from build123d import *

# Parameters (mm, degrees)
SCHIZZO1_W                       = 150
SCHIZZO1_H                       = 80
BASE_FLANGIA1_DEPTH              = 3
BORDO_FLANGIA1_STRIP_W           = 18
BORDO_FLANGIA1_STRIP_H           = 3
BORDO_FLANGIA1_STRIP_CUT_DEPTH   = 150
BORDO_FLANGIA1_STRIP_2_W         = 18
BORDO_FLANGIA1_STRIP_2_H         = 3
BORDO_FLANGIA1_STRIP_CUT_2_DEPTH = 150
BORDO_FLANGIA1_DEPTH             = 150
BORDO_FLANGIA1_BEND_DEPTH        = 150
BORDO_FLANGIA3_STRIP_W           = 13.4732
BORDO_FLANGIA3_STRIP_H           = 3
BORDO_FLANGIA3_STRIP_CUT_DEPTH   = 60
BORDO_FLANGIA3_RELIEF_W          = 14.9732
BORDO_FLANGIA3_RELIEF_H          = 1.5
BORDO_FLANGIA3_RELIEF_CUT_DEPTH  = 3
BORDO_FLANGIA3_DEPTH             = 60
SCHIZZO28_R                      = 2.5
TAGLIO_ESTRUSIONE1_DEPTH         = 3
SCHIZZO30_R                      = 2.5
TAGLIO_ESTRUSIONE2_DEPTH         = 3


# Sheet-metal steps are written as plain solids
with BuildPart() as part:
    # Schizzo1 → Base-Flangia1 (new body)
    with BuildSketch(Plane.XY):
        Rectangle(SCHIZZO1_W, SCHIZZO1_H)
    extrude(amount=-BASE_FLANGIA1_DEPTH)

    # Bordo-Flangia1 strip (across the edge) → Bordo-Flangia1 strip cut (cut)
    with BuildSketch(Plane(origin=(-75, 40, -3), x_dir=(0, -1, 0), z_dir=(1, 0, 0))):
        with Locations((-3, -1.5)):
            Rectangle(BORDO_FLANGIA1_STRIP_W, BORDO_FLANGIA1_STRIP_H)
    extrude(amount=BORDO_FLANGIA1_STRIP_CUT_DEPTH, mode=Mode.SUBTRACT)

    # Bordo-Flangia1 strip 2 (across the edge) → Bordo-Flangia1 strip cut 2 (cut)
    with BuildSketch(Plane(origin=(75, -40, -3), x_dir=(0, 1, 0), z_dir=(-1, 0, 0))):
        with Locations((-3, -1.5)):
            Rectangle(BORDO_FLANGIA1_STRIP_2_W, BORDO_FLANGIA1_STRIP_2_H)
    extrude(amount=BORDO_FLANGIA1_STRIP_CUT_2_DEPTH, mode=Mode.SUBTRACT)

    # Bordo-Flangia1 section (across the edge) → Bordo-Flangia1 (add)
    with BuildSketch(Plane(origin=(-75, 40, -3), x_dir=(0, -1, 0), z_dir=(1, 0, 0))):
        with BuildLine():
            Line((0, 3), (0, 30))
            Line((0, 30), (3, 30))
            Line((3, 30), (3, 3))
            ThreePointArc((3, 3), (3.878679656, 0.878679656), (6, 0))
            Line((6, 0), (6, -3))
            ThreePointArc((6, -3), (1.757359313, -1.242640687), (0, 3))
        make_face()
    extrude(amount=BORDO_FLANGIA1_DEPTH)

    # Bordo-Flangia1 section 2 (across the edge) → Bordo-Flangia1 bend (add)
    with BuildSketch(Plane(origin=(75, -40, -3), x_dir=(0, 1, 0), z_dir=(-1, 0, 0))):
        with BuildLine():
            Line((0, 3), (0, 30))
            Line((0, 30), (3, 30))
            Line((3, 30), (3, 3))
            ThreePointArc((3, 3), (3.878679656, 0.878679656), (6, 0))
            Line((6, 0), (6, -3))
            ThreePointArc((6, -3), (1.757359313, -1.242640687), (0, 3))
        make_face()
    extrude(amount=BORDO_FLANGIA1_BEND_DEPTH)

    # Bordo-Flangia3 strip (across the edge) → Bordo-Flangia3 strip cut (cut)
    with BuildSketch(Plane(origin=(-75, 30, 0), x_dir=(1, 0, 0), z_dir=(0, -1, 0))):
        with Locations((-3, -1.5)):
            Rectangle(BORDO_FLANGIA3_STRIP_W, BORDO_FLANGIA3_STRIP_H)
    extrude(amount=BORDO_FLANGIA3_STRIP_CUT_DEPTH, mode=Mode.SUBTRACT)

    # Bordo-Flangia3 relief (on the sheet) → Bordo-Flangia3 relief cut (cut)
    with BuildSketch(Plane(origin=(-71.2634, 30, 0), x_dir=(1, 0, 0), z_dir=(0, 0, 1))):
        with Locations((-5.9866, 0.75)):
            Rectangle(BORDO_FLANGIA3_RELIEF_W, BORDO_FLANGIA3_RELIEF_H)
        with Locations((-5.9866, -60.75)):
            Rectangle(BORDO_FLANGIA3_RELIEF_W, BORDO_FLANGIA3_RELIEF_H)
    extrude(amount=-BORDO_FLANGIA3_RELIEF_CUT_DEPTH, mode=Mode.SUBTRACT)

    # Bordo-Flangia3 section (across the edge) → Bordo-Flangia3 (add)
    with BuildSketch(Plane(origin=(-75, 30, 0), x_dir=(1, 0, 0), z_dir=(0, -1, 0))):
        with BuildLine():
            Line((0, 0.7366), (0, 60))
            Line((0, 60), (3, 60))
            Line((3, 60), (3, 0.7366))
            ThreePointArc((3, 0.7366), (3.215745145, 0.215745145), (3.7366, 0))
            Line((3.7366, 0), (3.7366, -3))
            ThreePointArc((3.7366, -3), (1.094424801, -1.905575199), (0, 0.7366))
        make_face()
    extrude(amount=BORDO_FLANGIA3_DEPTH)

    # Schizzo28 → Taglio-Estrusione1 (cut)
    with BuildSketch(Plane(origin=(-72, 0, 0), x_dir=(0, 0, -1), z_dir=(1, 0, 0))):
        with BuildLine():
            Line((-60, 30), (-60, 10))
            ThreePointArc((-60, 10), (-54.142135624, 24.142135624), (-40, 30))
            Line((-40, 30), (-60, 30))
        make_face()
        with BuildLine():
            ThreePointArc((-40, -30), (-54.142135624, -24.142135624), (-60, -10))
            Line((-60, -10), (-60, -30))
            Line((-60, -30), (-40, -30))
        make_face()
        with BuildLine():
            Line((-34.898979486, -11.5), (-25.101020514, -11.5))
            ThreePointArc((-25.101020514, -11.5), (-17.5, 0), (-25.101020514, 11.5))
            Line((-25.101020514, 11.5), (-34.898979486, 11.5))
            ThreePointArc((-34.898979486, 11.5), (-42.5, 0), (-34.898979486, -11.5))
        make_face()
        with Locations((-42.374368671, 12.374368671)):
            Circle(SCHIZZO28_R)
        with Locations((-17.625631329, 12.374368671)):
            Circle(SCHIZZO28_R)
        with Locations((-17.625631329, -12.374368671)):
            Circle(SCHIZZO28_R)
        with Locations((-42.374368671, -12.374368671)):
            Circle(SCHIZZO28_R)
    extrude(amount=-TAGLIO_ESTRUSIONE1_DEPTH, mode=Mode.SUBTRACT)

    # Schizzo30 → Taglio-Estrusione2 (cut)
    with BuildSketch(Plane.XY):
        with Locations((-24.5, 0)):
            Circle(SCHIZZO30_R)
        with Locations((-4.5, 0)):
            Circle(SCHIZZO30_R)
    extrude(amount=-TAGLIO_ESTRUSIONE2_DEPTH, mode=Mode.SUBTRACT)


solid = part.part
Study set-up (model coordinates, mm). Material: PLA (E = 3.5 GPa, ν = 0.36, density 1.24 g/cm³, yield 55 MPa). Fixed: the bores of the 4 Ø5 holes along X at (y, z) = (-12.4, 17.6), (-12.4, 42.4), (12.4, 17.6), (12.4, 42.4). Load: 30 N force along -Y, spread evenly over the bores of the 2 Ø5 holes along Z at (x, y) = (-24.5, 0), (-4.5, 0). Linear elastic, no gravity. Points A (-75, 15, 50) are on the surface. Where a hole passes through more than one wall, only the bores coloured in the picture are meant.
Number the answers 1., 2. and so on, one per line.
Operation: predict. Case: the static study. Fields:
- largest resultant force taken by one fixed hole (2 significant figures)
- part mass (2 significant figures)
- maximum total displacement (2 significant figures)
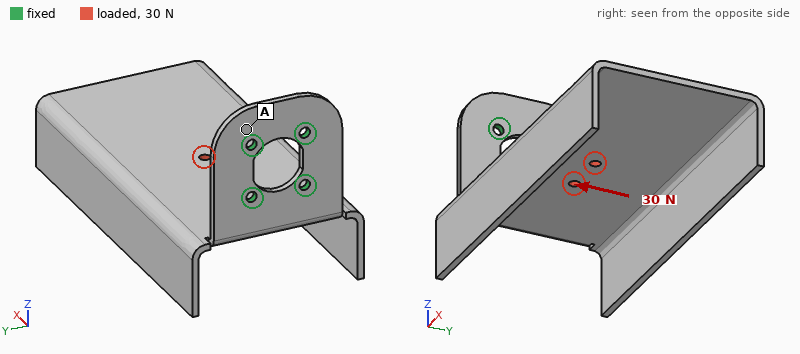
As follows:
1. 61 N
2. 86 g
3. 2.3 mm
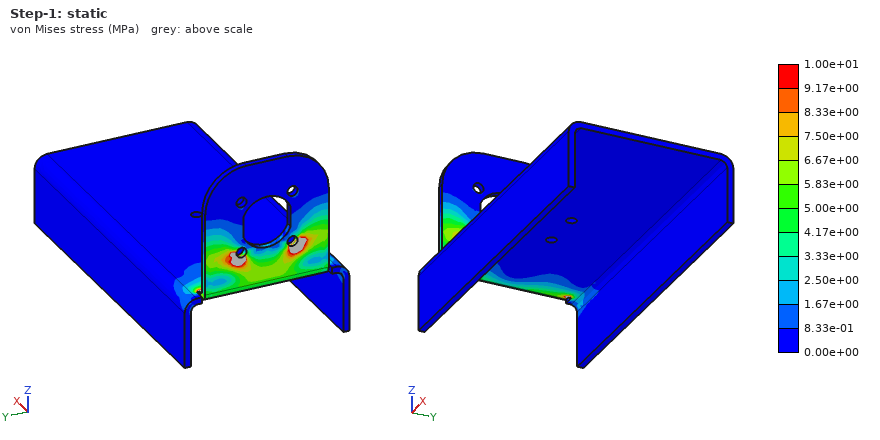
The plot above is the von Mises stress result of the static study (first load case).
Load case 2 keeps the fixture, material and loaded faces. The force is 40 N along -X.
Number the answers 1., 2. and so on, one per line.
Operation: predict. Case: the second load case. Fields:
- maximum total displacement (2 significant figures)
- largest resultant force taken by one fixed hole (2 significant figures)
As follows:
1. 2.3 mm
2. 22 N
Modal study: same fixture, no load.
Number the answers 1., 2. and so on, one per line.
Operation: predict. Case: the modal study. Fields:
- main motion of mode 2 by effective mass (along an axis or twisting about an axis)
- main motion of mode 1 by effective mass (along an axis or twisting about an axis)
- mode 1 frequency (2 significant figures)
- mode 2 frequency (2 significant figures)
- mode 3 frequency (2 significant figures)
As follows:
1. along Y
2. along Z
3. 27 Hz
4. 71 Hz
5. 90 Hz
